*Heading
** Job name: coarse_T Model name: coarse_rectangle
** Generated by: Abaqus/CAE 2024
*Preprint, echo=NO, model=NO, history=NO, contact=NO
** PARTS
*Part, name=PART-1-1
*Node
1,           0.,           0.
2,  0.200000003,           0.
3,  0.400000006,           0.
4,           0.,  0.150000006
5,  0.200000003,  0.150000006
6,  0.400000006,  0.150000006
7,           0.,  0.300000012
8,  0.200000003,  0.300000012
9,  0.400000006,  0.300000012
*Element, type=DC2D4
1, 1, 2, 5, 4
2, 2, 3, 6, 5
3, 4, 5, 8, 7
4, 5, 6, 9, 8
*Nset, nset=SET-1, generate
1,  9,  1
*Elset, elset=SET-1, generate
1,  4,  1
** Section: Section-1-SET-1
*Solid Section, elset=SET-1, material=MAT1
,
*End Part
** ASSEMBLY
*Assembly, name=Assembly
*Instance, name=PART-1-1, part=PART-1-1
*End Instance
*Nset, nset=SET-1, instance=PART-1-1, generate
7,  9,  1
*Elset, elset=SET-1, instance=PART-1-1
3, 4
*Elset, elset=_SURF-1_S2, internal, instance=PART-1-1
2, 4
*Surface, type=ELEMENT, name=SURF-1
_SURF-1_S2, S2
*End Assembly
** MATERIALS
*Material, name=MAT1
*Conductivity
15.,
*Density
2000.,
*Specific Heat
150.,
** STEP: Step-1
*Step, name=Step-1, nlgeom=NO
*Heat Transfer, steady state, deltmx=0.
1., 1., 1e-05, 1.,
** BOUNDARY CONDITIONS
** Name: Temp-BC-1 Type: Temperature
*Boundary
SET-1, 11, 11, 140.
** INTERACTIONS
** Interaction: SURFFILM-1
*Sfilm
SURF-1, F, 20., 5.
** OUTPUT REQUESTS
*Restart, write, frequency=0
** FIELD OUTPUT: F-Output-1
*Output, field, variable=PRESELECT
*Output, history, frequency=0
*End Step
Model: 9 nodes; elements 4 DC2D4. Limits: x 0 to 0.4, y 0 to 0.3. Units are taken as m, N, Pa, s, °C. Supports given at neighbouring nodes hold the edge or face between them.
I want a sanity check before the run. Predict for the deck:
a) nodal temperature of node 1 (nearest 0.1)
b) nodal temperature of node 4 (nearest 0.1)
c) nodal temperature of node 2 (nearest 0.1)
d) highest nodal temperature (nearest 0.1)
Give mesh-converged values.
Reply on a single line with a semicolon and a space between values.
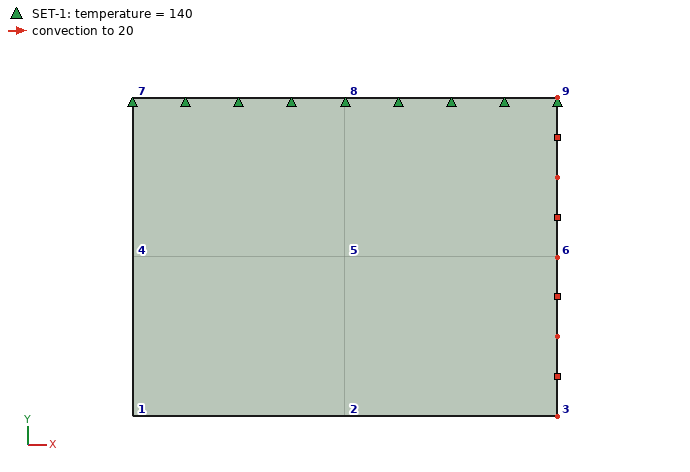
137.7 °C; 138.4 °C; 136.4 °C; 140.0 °C
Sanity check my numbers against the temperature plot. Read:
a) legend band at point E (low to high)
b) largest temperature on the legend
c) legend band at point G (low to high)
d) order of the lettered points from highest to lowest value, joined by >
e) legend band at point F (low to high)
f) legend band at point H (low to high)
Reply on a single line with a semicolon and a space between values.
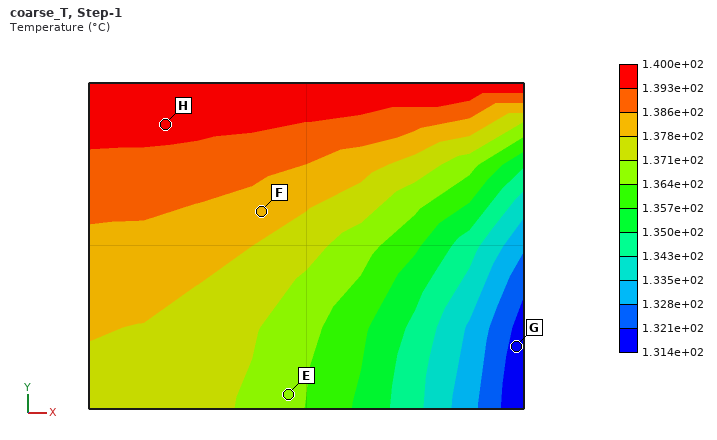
1.364e+02 to 1.371e+02 °C; 1.400e+02 °C; 1.314e+02 to 1.321e+02 °C; H > F > E > G; 1.378e+02 to 1.386e+02 °C; 1.393e+02 to 1.400e+02 °C
